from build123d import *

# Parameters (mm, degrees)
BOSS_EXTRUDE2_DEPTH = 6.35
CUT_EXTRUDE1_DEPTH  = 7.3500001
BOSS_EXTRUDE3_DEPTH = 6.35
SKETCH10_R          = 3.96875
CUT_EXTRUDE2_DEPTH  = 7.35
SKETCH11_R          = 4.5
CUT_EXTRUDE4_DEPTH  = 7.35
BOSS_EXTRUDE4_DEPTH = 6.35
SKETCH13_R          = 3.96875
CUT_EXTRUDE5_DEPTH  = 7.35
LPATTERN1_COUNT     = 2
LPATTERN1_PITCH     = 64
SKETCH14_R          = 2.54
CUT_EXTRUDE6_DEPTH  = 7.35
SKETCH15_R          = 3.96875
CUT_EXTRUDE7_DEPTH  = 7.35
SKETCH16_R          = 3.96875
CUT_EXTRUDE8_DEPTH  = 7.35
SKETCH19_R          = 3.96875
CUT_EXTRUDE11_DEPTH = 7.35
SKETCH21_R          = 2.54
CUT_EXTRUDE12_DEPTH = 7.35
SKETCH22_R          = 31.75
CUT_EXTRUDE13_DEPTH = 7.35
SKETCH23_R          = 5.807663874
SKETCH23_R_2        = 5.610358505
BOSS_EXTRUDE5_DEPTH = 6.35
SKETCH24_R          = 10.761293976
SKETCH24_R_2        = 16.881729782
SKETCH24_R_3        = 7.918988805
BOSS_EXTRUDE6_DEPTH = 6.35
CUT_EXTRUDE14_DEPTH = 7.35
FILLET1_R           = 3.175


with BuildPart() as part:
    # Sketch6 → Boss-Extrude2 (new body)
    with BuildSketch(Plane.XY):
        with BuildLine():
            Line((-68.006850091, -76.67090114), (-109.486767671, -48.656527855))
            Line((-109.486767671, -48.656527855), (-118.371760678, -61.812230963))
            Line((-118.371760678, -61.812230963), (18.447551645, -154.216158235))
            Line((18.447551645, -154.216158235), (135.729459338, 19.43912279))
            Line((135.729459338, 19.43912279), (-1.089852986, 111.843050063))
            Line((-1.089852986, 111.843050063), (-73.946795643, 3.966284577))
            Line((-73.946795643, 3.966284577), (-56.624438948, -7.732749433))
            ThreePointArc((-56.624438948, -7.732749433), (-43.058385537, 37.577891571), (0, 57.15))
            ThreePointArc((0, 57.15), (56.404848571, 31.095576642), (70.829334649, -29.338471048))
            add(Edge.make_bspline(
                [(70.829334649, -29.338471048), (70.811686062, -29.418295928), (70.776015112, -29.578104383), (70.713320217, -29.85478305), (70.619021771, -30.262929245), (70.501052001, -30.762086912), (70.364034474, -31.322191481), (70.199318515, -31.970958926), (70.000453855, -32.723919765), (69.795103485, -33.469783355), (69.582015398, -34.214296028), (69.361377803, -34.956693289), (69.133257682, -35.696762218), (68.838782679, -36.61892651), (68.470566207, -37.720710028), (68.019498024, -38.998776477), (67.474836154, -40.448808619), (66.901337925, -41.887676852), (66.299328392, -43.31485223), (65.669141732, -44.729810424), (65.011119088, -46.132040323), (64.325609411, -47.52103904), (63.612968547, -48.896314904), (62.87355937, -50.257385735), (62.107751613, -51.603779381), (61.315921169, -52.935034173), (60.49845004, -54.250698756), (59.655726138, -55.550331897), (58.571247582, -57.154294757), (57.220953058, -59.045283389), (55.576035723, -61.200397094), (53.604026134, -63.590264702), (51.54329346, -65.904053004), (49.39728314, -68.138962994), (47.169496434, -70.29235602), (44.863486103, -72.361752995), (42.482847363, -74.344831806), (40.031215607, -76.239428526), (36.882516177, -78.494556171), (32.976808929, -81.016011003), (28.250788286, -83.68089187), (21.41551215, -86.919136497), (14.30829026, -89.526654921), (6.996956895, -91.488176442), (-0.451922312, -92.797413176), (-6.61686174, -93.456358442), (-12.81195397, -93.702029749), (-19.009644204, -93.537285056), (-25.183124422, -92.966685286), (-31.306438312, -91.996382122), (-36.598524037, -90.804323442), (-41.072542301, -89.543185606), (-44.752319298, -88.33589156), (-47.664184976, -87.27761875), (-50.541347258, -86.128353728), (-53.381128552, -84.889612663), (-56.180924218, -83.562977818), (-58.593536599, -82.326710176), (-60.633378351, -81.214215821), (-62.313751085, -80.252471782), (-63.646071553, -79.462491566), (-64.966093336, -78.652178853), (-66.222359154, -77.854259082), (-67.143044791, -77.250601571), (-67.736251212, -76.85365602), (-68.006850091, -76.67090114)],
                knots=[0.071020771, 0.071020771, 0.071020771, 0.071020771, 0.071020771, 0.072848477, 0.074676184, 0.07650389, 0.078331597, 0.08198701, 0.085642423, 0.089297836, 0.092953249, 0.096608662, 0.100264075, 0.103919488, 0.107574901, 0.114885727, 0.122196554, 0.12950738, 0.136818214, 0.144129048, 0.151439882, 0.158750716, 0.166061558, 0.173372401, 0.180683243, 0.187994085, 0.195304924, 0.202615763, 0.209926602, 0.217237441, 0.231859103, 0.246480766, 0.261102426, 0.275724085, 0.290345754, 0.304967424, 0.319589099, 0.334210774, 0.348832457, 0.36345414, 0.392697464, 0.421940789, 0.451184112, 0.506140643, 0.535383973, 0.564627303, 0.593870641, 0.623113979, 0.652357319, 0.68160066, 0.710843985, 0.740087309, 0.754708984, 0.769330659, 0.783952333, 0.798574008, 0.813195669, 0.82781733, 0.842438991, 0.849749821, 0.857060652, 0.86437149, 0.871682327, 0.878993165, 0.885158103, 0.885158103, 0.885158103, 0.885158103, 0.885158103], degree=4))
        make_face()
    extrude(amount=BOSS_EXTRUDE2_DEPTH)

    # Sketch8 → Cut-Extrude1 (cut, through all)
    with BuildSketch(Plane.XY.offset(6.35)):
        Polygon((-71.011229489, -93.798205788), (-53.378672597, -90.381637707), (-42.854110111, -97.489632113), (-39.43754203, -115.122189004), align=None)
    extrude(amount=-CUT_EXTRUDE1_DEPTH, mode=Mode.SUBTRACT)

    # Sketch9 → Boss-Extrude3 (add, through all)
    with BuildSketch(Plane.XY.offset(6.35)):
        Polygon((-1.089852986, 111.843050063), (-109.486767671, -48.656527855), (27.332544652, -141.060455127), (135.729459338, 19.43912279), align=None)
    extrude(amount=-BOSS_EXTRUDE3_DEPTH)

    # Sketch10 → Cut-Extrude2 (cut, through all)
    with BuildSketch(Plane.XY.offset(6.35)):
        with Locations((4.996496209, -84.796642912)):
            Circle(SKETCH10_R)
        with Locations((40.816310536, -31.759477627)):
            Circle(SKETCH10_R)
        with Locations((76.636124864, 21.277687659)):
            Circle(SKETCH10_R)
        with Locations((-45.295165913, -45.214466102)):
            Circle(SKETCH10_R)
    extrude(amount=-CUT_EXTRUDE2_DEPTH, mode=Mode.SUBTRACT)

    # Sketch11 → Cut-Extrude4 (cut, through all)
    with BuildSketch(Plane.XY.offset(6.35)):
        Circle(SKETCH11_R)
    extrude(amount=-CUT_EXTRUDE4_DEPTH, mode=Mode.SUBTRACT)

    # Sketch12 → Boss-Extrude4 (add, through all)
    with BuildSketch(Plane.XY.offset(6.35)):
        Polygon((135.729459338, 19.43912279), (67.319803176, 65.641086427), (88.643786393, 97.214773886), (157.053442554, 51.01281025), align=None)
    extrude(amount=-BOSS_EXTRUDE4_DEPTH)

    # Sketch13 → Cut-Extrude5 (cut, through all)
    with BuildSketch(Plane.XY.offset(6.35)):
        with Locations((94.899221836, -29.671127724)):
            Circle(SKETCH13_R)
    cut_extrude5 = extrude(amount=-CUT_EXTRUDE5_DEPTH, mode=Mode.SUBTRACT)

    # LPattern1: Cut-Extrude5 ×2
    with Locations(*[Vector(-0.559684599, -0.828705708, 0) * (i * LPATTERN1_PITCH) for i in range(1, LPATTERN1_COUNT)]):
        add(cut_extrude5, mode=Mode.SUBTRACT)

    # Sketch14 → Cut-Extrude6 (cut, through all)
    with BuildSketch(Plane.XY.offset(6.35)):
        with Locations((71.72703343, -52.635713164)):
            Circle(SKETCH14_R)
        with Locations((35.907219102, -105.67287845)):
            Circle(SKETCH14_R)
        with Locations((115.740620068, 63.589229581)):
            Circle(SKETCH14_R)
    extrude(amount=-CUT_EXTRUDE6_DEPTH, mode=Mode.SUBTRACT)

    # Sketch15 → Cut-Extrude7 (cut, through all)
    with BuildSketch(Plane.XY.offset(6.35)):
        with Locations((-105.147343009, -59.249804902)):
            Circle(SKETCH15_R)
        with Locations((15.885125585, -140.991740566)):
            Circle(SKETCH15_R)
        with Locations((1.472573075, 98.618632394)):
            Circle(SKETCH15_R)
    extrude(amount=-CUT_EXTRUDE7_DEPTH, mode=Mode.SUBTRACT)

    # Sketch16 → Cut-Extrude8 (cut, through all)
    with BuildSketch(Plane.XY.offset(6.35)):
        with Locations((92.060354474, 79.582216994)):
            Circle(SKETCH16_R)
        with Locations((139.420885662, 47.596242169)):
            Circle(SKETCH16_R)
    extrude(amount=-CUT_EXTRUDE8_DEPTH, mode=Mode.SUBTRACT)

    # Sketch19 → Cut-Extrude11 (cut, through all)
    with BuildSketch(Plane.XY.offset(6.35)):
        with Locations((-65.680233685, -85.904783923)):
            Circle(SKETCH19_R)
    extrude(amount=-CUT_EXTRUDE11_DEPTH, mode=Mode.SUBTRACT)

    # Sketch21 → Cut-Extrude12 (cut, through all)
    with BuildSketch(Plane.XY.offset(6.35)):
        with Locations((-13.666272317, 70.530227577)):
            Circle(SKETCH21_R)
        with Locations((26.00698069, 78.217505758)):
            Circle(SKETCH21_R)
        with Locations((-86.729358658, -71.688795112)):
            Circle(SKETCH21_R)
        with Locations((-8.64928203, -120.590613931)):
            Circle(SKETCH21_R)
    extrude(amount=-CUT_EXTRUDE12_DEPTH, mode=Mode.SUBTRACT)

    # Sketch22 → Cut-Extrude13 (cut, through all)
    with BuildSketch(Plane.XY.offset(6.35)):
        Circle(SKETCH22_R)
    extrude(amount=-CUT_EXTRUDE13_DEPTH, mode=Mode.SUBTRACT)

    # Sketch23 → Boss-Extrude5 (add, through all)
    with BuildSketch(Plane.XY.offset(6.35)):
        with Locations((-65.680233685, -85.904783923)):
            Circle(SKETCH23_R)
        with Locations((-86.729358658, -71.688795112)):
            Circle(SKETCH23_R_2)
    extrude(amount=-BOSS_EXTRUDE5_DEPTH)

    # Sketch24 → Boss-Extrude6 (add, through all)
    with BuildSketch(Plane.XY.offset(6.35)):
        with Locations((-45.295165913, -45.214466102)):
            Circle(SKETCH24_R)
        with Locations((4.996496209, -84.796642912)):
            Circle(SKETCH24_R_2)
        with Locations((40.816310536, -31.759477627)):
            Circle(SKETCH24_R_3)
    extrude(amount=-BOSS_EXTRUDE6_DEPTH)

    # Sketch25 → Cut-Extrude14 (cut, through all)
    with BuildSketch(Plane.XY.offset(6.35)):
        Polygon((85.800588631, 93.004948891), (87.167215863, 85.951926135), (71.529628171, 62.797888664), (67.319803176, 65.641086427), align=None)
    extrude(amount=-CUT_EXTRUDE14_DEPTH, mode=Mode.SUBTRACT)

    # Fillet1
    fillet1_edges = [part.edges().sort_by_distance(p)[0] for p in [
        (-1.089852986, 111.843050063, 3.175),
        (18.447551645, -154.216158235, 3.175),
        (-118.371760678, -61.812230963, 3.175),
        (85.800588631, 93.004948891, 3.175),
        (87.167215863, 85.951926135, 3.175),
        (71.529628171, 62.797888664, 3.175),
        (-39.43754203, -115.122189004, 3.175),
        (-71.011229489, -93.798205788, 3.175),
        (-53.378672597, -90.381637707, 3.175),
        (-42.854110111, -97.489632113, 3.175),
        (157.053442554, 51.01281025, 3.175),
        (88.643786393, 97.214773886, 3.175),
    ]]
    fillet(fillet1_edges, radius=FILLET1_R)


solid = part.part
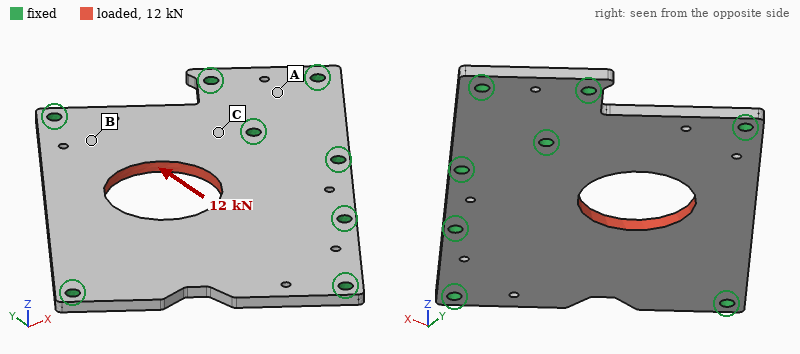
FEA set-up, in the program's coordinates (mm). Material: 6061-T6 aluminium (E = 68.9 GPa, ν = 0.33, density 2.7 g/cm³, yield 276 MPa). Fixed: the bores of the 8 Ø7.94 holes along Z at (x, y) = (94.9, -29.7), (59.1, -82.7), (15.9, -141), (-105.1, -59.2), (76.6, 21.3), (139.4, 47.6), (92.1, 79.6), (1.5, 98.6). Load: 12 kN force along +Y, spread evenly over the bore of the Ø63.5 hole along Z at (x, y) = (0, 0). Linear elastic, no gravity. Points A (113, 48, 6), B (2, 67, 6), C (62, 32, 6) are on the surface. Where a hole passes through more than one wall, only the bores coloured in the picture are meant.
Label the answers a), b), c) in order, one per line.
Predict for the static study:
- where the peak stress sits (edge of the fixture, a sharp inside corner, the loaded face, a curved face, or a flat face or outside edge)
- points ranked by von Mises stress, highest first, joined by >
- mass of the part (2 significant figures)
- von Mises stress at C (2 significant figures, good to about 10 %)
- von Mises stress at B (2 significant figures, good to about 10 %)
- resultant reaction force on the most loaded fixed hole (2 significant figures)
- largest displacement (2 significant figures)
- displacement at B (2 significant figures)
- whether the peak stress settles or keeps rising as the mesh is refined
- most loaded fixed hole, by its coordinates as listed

a) edge of the fixture
b) B > C > A
c) 580 g
d) 8.0 MPa
e) 13 MPa
f) 3.4 kN
g) 23 µm
h) 7.9 µm
i) keeps rising
j) (1.5, 98.6)
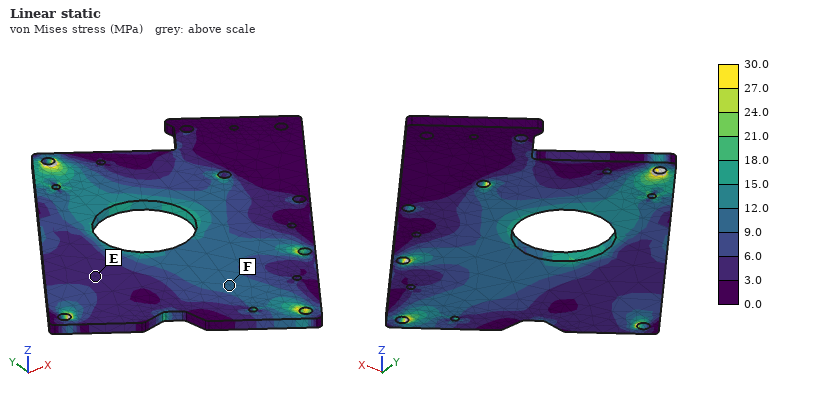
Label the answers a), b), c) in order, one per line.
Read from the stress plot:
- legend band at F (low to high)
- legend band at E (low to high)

a) 9.0 to 12.0 MPa
b) 3.0 to 6.0 MPa
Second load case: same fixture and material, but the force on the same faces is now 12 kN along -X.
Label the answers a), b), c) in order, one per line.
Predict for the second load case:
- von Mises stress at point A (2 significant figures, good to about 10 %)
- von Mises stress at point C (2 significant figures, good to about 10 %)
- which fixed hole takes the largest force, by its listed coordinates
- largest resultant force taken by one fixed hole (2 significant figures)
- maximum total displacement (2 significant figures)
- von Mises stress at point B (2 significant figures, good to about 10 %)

a) 4.1 MPa
b) 12 MPa
c) (76.6, 21.3)
d) 3.3 kN
e) 28 µm
f) 3.1 MPa
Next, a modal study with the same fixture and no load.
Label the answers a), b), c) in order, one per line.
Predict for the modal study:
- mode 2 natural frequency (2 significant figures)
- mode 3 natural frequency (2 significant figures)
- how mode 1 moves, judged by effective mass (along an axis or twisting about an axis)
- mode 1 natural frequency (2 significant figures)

a) 1500 Hz
b) 2300 Hz
c) along Z
d) 960 Hz
